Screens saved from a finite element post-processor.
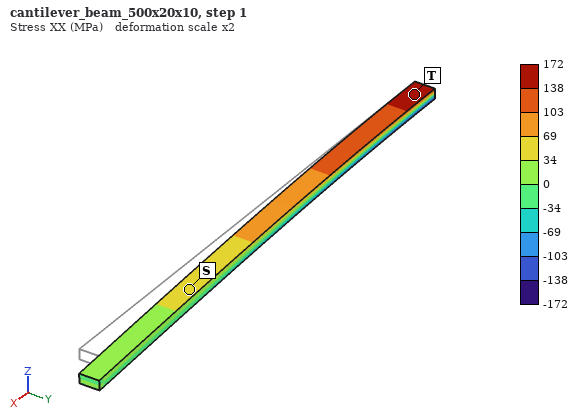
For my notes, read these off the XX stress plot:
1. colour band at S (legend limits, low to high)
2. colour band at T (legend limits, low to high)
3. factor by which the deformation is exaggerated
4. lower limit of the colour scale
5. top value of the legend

34 to 69 MPa
138 to 172 MPa
2
-172 MPa
172 MPa
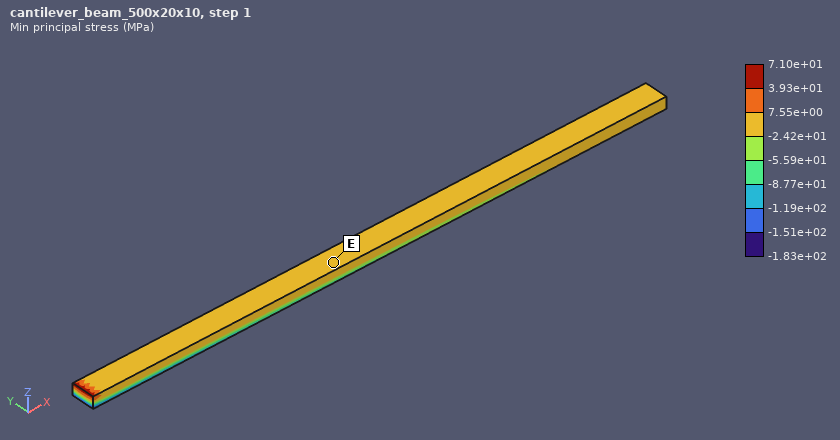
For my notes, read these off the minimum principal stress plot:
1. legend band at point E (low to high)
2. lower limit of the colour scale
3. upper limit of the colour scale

-2.42e+01 to 7.55e+00 MPa
-1.83e+02 MPa
7.10e+01 MPa
